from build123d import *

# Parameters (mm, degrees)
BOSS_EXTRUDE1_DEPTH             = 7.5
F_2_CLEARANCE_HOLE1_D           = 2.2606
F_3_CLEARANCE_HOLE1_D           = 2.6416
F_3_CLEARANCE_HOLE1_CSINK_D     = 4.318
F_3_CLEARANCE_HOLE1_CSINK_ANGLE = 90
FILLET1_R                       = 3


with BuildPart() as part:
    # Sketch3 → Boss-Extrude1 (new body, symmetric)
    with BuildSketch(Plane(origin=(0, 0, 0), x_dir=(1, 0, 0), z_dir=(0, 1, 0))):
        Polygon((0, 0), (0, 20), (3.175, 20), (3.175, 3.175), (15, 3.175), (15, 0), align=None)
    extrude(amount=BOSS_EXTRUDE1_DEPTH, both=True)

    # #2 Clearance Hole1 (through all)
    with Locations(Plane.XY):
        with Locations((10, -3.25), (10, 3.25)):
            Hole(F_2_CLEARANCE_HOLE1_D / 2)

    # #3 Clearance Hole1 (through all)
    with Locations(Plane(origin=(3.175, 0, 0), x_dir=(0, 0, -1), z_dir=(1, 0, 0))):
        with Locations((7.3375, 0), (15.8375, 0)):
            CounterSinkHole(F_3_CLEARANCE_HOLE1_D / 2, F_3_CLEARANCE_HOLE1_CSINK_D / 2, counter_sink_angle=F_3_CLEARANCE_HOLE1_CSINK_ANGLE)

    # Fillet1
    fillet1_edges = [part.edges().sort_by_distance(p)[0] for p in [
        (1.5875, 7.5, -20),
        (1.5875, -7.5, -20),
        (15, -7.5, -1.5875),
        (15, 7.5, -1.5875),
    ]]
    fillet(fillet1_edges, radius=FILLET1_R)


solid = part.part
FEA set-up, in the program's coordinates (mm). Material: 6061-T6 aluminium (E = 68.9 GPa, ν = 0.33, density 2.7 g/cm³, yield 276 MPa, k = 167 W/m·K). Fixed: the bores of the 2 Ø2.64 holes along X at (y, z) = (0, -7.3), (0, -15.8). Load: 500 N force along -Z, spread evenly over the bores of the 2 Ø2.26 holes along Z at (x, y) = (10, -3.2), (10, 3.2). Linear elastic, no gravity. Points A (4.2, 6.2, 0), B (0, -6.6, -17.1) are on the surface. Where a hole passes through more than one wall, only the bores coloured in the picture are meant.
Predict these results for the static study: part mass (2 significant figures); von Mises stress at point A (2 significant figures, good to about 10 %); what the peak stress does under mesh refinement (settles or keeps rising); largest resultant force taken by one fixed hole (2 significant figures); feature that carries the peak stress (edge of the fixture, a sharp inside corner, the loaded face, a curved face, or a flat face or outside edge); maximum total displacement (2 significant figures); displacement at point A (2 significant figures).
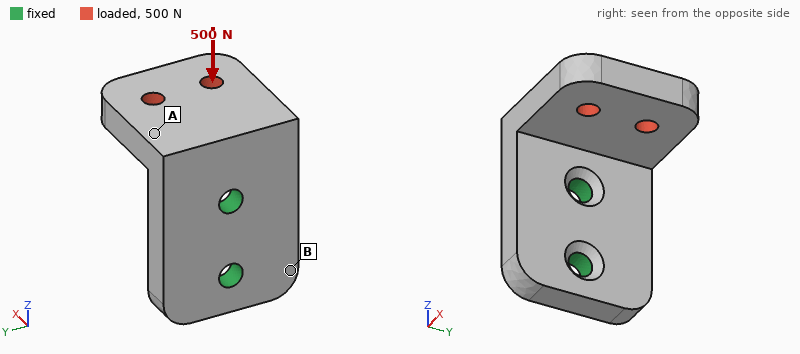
3.8 g
110 MPa
keeps rising
370 N
edge of the fixture
0.20 mm
0.060 mm
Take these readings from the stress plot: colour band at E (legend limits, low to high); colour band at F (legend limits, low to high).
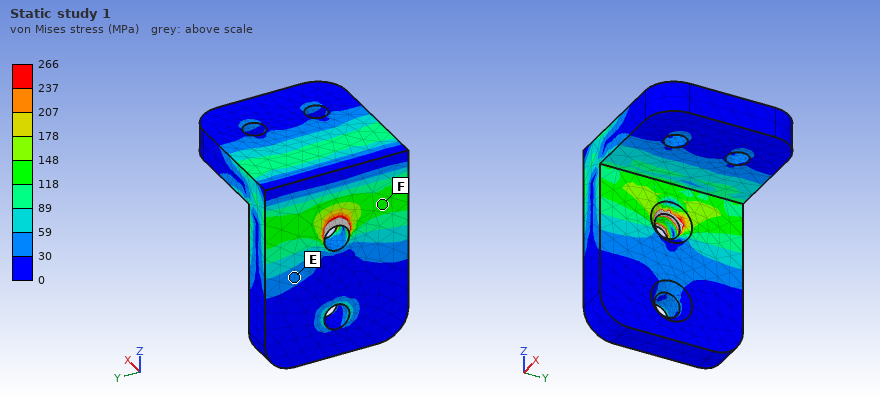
30 to 59 MPa
118 to 148 MPa
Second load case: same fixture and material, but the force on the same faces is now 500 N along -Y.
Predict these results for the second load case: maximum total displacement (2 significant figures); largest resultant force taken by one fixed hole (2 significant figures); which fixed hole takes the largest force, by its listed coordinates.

0.11 mm
700 N
(0, -7.3)
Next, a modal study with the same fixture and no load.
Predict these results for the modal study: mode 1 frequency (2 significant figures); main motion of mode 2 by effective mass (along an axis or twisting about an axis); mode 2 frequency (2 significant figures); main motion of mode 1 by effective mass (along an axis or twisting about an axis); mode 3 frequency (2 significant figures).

8500 Hz
along Y
10 kHz
along Z
25 kHz
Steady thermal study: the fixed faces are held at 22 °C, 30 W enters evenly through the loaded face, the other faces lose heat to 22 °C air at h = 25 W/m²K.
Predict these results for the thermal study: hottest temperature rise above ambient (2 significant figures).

58 K
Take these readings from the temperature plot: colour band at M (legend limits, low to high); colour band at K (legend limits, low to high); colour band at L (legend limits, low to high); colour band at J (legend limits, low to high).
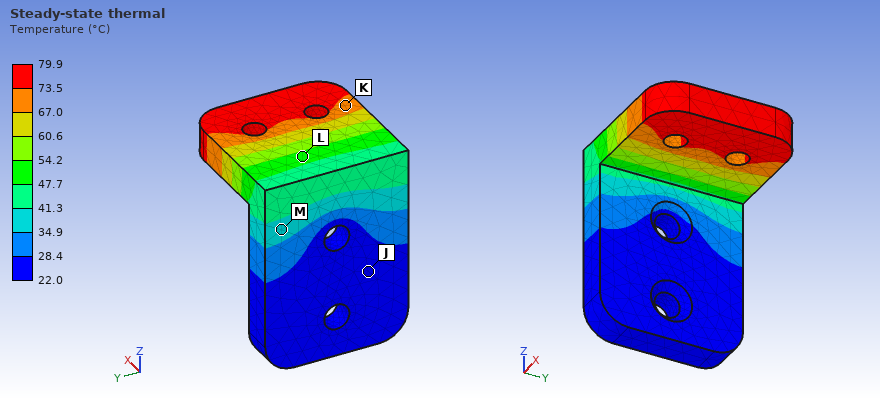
34.9 to 41.3 °C
67.0 to 73.5 °C
47.7 to 54.2 °C
22.0 to 28.4 °C
